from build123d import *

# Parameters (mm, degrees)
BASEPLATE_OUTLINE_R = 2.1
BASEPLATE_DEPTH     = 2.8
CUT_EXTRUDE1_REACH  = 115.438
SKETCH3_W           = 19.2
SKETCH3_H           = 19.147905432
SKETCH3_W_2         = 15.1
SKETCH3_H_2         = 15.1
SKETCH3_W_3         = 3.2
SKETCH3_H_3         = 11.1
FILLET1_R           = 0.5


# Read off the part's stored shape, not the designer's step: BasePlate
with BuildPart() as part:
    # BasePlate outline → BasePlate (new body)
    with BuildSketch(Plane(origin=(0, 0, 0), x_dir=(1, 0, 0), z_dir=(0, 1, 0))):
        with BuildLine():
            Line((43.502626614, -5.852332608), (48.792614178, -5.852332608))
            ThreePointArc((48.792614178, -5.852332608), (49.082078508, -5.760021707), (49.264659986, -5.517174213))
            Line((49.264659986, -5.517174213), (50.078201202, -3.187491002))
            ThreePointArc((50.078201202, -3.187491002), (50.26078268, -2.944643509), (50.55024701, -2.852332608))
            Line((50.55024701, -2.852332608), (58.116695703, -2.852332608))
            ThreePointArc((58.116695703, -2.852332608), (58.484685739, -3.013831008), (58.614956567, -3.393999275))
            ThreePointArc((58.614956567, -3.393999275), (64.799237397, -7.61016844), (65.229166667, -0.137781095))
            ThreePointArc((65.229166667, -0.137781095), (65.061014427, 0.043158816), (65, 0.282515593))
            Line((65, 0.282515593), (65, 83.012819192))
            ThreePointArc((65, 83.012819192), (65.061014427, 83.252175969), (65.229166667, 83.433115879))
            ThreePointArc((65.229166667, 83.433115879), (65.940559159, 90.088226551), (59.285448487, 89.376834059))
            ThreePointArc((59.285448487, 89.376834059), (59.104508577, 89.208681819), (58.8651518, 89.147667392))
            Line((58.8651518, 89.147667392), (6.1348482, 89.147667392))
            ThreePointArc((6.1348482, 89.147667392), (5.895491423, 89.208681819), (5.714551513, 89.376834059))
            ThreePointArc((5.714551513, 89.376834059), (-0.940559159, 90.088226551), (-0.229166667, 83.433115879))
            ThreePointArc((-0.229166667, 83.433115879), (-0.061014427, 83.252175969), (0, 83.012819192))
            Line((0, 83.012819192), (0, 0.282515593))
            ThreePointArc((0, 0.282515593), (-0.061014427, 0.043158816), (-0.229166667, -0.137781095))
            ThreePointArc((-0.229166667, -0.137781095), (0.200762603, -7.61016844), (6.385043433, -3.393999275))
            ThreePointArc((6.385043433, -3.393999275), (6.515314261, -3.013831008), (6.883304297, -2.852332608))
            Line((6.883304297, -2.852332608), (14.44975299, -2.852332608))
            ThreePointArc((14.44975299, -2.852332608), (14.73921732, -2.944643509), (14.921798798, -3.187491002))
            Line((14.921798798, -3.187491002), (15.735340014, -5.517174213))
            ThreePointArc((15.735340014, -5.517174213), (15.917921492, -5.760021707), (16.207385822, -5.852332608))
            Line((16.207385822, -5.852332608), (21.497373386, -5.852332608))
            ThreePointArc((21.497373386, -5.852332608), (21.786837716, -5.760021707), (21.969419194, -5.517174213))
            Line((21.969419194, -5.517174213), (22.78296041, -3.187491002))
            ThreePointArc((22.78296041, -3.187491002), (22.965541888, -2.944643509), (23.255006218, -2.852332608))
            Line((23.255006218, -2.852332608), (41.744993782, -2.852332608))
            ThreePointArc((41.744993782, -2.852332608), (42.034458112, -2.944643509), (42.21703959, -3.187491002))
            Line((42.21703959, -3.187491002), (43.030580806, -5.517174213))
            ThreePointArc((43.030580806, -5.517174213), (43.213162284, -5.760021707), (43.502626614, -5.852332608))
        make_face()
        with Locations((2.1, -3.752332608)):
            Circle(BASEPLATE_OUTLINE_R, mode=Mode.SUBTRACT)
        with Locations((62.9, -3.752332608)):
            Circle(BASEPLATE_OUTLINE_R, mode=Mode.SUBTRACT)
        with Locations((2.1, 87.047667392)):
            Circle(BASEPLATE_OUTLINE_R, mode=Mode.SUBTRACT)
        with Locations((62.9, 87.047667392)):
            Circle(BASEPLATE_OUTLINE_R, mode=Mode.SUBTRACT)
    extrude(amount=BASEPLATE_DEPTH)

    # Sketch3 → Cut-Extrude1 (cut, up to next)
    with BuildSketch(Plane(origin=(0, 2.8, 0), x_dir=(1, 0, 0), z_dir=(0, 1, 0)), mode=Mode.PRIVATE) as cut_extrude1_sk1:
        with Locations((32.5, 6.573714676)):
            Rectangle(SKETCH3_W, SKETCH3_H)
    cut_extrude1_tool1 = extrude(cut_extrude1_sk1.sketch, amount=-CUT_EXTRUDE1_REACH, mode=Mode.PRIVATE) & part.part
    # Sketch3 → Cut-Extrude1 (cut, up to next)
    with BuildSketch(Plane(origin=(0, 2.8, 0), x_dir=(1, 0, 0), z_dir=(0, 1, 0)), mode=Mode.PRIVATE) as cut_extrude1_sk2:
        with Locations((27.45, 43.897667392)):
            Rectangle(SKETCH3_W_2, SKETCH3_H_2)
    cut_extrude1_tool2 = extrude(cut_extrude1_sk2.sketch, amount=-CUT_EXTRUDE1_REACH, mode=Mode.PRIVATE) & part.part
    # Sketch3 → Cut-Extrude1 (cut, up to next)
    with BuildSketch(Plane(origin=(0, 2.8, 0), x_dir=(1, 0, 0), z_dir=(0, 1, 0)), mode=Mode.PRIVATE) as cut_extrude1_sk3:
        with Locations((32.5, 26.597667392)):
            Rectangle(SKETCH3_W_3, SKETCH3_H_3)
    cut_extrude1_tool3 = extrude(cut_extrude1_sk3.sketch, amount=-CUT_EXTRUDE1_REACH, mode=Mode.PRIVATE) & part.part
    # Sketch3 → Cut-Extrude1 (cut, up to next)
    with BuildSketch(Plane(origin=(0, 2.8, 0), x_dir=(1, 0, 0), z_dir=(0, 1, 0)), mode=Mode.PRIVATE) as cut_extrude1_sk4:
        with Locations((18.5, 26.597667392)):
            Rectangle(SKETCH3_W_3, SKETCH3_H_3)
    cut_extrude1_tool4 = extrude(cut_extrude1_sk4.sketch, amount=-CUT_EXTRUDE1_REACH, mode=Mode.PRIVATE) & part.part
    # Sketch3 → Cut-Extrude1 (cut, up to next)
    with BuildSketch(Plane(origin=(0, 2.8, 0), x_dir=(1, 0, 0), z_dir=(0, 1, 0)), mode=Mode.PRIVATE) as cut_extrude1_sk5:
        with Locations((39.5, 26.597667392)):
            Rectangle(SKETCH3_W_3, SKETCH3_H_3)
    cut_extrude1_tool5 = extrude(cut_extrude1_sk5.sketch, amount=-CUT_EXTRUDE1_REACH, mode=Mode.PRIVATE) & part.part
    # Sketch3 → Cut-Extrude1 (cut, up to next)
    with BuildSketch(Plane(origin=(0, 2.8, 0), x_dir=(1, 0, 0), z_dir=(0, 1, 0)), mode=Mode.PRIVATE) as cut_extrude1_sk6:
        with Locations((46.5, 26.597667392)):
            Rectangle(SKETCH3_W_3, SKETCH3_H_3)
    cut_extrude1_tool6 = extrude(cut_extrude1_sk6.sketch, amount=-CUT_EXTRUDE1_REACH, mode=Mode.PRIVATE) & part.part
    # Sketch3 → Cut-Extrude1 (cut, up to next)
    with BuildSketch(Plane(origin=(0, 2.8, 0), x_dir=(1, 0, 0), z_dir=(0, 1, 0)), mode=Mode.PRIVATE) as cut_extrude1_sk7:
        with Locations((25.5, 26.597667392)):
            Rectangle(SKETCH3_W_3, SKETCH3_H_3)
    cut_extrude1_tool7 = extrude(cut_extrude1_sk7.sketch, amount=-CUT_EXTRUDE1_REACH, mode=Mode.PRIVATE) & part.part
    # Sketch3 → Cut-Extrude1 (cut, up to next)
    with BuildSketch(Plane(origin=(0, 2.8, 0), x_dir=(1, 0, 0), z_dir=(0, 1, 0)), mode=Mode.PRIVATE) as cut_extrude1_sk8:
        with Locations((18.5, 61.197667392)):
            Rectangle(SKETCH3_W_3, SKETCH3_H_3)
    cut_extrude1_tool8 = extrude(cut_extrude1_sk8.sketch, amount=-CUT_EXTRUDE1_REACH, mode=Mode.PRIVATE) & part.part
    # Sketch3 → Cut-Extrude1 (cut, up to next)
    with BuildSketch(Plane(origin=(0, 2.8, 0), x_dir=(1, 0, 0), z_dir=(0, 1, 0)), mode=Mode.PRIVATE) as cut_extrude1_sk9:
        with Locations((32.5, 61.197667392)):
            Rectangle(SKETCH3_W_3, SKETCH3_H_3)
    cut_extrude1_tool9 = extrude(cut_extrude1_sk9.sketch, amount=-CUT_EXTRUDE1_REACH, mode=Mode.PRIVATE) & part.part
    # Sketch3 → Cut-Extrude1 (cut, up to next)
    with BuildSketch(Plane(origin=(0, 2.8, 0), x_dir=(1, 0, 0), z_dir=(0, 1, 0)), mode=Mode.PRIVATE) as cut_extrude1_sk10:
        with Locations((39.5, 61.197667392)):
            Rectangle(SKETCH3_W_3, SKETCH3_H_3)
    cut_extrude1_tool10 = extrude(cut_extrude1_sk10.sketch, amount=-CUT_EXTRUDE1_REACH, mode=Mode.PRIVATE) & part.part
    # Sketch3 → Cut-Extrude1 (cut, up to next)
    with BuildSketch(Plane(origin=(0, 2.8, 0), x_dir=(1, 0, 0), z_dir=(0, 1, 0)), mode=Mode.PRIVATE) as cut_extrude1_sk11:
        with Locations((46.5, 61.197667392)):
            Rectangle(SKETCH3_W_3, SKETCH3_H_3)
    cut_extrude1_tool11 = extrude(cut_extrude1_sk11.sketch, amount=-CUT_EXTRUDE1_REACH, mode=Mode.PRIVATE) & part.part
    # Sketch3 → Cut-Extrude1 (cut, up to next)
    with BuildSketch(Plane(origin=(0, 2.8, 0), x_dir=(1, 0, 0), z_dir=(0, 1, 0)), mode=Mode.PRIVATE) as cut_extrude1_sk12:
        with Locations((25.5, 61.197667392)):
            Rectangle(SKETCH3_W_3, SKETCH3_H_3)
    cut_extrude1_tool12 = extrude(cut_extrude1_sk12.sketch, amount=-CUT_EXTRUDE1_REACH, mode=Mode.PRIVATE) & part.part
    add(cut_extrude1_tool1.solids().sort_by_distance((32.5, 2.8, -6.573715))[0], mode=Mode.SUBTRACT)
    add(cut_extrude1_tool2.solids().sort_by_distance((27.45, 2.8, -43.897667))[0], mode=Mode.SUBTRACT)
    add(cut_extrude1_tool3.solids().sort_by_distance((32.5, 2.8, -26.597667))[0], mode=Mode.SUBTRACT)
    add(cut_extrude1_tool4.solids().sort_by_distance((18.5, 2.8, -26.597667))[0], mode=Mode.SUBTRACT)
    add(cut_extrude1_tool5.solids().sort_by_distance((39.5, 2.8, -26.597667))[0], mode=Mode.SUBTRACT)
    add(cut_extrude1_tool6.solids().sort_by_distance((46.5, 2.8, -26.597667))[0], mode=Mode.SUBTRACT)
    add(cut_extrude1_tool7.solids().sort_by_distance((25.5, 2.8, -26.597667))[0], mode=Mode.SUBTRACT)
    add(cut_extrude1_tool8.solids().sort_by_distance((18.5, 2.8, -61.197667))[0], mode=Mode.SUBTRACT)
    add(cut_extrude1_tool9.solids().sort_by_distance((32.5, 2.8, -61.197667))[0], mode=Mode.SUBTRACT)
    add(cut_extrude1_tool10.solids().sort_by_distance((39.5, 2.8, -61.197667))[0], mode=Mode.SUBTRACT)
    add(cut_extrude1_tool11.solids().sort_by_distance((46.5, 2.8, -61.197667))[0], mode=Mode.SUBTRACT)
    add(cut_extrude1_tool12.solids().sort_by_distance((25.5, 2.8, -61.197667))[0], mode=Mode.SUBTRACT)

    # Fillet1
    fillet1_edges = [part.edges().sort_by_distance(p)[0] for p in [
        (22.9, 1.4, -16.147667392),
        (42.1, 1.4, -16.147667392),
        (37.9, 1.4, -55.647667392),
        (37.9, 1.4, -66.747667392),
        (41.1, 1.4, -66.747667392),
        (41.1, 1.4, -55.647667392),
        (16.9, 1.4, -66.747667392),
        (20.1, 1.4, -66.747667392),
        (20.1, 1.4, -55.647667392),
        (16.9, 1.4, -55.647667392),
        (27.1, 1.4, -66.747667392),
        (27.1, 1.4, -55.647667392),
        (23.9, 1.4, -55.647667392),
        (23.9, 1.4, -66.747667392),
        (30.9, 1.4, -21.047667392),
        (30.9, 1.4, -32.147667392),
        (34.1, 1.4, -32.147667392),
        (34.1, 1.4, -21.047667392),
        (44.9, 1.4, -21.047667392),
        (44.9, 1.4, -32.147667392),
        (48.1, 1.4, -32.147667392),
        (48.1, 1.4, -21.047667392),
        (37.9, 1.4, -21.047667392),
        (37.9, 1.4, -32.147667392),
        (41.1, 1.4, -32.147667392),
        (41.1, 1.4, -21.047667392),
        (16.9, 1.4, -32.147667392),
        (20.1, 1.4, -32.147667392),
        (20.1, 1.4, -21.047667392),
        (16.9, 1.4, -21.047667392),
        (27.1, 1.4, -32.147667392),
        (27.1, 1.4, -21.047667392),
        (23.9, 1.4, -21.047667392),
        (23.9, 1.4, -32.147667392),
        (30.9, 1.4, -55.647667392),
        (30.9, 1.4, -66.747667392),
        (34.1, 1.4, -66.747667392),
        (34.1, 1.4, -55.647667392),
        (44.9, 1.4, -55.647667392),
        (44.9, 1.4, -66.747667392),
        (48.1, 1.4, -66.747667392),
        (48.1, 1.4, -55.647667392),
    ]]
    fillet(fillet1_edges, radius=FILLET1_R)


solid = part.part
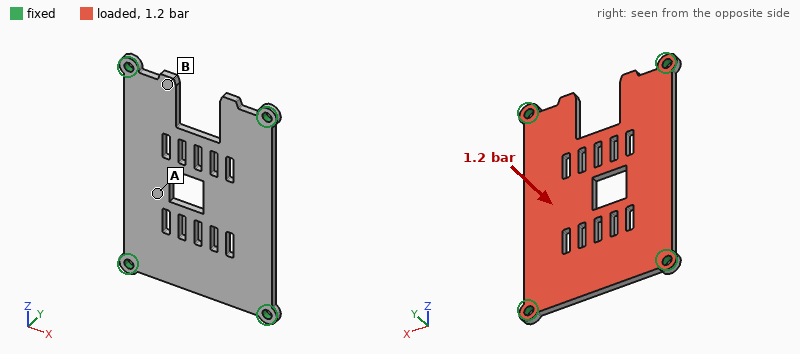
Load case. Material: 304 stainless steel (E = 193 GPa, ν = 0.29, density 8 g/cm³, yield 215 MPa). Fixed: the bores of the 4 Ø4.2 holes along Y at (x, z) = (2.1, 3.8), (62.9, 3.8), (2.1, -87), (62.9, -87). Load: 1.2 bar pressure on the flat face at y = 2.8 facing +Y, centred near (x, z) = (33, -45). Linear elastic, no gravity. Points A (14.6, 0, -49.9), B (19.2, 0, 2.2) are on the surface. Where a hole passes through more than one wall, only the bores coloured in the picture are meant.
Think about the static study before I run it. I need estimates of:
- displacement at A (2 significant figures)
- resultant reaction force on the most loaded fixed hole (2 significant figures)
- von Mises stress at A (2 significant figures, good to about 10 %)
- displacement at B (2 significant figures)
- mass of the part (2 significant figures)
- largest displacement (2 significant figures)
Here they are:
0.10 mm
170 N
38 MPa
0.019 mm
120 g
0.12 mm
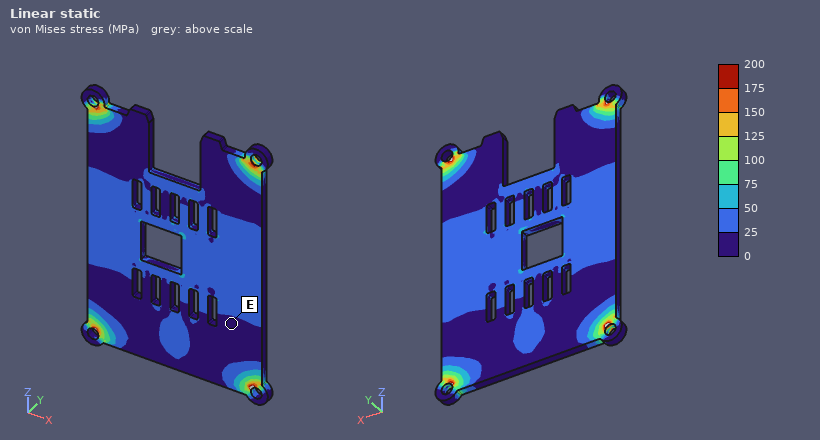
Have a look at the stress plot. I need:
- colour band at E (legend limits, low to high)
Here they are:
0 to 25 MPa
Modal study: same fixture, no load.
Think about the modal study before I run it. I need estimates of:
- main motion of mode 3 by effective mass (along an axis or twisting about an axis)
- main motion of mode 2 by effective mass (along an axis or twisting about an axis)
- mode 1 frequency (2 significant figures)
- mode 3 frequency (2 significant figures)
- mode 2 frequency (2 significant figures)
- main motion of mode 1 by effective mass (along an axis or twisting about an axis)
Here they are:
twisting about X
twisting about Z
1300 Hz
3200 Hz
2100 Hz
along Y
